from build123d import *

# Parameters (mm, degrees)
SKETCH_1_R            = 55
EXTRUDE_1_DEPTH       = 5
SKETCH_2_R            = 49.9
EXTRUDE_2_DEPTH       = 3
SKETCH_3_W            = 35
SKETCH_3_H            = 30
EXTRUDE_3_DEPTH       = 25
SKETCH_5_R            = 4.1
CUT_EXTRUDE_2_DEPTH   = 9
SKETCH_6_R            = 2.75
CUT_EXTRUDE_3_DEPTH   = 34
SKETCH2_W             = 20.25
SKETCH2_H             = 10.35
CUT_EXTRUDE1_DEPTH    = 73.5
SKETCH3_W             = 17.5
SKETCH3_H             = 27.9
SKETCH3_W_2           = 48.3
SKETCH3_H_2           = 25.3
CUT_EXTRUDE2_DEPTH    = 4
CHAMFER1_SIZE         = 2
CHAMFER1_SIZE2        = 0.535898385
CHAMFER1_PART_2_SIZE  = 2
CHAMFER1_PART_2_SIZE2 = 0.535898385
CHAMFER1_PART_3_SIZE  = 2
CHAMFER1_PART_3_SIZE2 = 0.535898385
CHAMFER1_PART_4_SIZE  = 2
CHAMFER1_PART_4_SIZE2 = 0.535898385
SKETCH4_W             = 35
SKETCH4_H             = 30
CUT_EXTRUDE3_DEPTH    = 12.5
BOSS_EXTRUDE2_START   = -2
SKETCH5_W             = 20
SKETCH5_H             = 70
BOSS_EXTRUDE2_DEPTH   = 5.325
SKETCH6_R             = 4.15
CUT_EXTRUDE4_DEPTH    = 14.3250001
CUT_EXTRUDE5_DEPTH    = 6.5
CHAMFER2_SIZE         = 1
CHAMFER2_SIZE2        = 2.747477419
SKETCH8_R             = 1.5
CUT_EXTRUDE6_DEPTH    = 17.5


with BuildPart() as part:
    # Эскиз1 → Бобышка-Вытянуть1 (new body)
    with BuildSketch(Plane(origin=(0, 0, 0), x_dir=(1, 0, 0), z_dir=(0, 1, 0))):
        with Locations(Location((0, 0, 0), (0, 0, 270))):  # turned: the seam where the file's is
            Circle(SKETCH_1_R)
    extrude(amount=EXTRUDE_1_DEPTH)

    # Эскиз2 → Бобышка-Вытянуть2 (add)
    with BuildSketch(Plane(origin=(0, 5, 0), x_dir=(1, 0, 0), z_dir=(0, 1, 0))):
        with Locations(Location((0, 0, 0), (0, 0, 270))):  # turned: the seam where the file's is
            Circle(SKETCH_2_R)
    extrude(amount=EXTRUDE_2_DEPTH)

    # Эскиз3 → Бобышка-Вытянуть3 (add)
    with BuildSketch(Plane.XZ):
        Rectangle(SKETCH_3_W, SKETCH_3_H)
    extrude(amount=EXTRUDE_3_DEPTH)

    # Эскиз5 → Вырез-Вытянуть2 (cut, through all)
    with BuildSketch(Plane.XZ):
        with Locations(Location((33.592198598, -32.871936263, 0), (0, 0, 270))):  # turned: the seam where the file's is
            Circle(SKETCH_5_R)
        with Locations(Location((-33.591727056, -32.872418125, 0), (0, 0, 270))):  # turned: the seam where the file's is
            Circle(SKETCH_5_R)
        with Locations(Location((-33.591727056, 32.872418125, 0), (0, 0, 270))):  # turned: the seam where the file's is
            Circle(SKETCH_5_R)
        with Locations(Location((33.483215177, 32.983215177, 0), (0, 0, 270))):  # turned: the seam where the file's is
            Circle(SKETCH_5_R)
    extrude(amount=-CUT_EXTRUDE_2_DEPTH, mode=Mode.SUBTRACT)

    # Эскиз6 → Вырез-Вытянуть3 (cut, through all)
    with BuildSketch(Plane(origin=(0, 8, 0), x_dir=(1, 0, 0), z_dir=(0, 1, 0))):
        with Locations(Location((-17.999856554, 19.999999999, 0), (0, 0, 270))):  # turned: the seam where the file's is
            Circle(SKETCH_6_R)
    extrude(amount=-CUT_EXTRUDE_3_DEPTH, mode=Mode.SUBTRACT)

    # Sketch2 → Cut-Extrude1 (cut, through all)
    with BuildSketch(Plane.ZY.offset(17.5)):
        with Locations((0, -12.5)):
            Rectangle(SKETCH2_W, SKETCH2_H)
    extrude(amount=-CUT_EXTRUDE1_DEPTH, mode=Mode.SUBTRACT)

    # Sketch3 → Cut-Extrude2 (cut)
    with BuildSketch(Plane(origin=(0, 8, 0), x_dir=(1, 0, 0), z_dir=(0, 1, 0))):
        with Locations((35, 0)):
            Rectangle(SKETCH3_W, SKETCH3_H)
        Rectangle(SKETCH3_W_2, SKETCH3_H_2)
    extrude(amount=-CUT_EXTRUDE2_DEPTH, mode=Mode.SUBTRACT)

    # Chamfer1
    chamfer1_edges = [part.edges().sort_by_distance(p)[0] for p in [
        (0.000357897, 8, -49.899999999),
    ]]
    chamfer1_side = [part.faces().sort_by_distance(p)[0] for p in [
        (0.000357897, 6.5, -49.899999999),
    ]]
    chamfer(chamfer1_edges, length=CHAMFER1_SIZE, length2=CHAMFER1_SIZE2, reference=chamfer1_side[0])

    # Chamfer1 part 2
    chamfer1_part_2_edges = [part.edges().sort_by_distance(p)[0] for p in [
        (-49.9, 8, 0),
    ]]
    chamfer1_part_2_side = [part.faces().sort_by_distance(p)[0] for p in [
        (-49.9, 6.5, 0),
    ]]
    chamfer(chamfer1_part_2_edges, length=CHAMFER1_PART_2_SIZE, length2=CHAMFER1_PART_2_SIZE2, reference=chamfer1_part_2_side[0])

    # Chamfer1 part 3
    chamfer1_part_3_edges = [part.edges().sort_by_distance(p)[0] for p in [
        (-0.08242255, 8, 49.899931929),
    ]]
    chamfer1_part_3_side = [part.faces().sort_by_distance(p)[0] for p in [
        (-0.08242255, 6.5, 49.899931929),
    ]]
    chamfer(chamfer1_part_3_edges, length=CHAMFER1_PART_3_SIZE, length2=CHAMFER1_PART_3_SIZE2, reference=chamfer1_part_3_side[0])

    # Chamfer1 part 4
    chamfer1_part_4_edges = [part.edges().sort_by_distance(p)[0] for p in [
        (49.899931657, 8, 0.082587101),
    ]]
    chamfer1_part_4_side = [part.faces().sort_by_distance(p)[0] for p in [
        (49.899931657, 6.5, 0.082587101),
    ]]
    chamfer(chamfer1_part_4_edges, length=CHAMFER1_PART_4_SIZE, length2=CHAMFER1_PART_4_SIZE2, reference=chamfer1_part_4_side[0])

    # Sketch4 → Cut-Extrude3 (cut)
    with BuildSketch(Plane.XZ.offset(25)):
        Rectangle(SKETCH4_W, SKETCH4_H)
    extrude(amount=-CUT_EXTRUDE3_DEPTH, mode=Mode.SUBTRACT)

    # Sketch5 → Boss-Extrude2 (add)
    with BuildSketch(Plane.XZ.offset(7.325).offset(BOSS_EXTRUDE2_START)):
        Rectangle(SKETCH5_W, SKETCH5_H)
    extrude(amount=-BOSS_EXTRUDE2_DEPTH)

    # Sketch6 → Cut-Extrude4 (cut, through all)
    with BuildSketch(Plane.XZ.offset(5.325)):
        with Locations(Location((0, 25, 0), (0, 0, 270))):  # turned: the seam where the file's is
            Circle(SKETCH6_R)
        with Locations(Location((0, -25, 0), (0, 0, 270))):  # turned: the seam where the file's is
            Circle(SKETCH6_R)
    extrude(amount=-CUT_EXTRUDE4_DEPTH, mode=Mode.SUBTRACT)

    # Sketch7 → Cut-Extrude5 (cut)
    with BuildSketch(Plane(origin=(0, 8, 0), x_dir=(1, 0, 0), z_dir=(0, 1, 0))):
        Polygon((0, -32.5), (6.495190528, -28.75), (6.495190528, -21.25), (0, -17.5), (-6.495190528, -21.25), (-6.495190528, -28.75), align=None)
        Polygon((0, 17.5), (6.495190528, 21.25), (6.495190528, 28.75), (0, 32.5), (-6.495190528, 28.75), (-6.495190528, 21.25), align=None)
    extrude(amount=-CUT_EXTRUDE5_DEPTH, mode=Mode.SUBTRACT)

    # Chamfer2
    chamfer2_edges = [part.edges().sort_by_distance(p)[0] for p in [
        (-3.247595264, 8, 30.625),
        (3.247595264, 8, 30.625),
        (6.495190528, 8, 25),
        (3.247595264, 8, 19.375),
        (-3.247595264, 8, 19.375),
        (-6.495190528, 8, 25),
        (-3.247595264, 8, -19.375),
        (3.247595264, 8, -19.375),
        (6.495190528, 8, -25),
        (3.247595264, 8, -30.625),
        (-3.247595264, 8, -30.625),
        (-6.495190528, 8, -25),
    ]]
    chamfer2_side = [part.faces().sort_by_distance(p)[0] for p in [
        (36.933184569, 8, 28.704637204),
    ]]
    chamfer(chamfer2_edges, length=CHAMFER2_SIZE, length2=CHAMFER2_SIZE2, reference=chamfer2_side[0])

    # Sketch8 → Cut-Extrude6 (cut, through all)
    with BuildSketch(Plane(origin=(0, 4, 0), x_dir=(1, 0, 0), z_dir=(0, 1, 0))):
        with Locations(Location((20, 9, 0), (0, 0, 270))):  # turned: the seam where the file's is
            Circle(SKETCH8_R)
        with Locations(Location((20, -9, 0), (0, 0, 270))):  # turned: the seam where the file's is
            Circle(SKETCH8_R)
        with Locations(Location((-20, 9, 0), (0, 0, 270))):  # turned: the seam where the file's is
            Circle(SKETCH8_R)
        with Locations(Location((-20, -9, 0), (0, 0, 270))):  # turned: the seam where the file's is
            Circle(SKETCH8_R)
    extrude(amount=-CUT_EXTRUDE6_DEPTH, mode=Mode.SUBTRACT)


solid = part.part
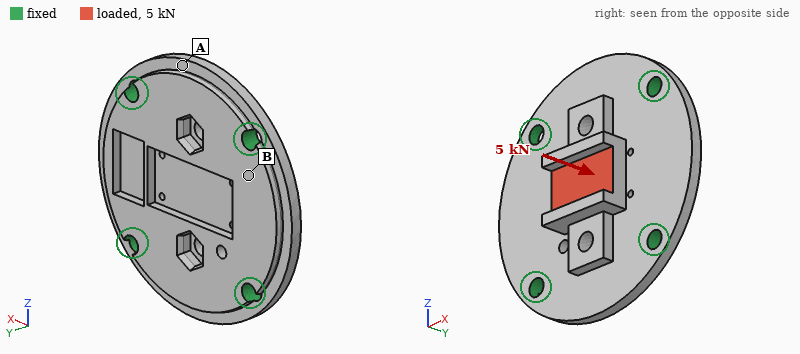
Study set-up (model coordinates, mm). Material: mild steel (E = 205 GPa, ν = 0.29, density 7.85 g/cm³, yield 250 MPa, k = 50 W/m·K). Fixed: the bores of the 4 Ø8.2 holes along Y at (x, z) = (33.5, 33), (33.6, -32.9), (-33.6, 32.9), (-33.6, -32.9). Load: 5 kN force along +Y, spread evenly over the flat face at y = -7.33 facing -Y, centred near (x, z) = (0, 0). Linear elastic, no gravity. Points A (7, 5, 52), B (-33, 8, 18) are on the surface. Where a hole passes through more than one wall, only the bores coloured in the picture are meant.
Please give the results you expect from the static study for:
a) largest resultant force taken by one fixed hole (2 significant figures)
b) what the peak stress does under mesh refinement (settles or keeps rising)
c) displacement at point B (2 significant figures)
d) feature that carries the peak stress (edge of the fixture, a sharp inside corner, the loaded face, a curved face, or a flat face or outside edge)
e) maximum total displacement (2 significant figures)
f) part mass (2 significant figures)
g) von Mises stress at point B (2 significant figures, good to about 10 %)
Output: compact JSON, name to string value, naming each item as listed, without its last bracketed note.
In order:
{"largest resultant force taken by one fixed hole": "2.0 kN", "what the peak stress does under mesh refinement": "keeps rising", "displacement at point B": "4.0 µm", "feature that carries the peak stress": "edge of the fixture", "maximum total displacement": "17 µm", "part mass": "570 g", "von Mises stress at point B": "20 MPa"}
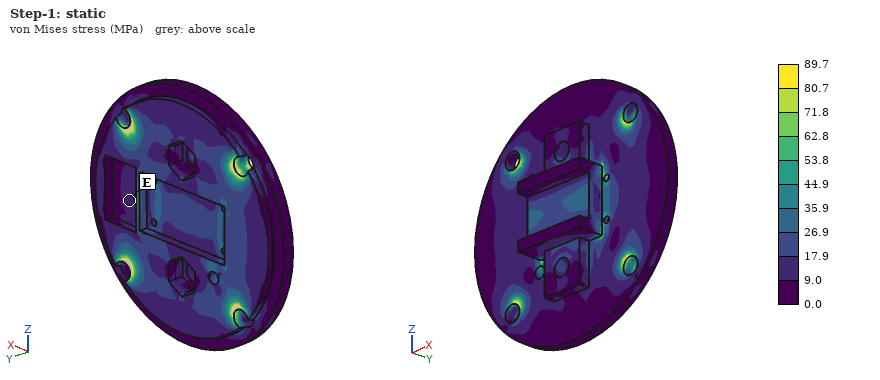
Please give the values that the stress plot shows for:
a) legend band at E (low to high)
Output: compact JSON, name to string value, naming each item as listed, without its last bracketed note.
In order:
{"legend band at E": "9.0 to 17.9 MPa"}
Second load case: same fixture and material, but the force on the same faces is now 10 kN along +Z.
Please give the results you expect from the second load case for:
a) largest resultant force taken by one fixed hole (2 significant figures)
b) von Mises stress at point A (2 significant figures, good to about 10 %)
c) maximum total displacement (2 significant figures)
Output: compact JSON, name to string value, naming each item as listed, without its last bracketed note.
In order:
{"largest resultant force taken by one fixed hole": "2.9 kN", "von Mises stress at point A": "15 MPa", "maximum total displacement": "10.0 µm"}
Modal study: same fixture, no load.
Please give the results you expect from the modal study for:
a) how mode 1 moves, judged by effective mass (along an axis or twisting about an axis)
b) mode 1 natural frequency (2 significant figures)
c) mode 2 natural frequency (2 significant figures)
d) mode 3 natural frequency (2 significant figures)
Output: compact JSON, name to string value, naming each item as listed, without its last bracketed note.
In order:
{"how mode 1 moves, judged by effective mass": "along Y", "mode 1 natural frequency": "6500 Hz", "mode 2 natural frequency": "7900 Hz", "mode 3 natural frequency": "8200 Hz"}
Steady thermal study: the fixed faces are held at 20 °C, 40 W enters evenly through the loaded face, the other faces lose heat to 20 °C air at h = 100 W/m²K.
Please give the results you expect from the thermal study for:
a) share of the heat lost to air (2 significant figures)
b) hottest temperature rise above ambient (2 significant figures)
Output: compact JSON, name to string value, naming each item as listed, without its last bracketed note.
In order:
{"share of the heat lost to air": "46 %", "hottest temperature rise above ambient": "29 K"}
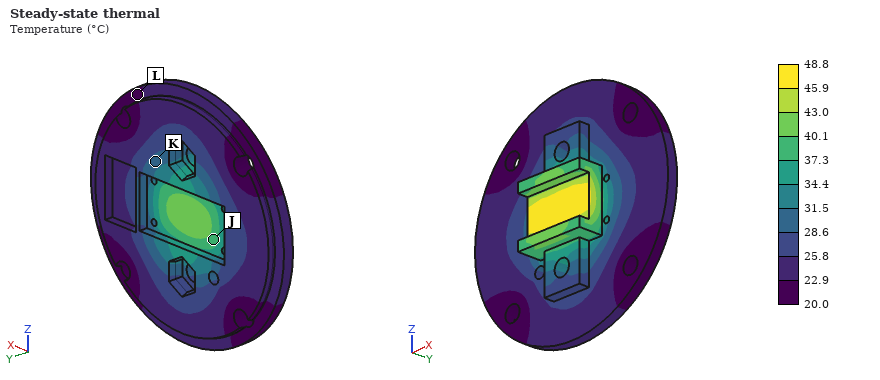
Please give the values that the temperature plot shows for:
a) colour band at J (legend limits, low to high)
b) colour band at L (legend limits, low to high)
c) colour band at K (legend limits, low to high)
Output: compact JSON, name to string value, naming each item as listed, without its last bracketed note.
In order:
{"colour band at J": "37.3 to 40.1 °C", "colour band at L": "20.0 to 22.9 °C", "colour band at K": "28.6 to 31.5 °C"}
